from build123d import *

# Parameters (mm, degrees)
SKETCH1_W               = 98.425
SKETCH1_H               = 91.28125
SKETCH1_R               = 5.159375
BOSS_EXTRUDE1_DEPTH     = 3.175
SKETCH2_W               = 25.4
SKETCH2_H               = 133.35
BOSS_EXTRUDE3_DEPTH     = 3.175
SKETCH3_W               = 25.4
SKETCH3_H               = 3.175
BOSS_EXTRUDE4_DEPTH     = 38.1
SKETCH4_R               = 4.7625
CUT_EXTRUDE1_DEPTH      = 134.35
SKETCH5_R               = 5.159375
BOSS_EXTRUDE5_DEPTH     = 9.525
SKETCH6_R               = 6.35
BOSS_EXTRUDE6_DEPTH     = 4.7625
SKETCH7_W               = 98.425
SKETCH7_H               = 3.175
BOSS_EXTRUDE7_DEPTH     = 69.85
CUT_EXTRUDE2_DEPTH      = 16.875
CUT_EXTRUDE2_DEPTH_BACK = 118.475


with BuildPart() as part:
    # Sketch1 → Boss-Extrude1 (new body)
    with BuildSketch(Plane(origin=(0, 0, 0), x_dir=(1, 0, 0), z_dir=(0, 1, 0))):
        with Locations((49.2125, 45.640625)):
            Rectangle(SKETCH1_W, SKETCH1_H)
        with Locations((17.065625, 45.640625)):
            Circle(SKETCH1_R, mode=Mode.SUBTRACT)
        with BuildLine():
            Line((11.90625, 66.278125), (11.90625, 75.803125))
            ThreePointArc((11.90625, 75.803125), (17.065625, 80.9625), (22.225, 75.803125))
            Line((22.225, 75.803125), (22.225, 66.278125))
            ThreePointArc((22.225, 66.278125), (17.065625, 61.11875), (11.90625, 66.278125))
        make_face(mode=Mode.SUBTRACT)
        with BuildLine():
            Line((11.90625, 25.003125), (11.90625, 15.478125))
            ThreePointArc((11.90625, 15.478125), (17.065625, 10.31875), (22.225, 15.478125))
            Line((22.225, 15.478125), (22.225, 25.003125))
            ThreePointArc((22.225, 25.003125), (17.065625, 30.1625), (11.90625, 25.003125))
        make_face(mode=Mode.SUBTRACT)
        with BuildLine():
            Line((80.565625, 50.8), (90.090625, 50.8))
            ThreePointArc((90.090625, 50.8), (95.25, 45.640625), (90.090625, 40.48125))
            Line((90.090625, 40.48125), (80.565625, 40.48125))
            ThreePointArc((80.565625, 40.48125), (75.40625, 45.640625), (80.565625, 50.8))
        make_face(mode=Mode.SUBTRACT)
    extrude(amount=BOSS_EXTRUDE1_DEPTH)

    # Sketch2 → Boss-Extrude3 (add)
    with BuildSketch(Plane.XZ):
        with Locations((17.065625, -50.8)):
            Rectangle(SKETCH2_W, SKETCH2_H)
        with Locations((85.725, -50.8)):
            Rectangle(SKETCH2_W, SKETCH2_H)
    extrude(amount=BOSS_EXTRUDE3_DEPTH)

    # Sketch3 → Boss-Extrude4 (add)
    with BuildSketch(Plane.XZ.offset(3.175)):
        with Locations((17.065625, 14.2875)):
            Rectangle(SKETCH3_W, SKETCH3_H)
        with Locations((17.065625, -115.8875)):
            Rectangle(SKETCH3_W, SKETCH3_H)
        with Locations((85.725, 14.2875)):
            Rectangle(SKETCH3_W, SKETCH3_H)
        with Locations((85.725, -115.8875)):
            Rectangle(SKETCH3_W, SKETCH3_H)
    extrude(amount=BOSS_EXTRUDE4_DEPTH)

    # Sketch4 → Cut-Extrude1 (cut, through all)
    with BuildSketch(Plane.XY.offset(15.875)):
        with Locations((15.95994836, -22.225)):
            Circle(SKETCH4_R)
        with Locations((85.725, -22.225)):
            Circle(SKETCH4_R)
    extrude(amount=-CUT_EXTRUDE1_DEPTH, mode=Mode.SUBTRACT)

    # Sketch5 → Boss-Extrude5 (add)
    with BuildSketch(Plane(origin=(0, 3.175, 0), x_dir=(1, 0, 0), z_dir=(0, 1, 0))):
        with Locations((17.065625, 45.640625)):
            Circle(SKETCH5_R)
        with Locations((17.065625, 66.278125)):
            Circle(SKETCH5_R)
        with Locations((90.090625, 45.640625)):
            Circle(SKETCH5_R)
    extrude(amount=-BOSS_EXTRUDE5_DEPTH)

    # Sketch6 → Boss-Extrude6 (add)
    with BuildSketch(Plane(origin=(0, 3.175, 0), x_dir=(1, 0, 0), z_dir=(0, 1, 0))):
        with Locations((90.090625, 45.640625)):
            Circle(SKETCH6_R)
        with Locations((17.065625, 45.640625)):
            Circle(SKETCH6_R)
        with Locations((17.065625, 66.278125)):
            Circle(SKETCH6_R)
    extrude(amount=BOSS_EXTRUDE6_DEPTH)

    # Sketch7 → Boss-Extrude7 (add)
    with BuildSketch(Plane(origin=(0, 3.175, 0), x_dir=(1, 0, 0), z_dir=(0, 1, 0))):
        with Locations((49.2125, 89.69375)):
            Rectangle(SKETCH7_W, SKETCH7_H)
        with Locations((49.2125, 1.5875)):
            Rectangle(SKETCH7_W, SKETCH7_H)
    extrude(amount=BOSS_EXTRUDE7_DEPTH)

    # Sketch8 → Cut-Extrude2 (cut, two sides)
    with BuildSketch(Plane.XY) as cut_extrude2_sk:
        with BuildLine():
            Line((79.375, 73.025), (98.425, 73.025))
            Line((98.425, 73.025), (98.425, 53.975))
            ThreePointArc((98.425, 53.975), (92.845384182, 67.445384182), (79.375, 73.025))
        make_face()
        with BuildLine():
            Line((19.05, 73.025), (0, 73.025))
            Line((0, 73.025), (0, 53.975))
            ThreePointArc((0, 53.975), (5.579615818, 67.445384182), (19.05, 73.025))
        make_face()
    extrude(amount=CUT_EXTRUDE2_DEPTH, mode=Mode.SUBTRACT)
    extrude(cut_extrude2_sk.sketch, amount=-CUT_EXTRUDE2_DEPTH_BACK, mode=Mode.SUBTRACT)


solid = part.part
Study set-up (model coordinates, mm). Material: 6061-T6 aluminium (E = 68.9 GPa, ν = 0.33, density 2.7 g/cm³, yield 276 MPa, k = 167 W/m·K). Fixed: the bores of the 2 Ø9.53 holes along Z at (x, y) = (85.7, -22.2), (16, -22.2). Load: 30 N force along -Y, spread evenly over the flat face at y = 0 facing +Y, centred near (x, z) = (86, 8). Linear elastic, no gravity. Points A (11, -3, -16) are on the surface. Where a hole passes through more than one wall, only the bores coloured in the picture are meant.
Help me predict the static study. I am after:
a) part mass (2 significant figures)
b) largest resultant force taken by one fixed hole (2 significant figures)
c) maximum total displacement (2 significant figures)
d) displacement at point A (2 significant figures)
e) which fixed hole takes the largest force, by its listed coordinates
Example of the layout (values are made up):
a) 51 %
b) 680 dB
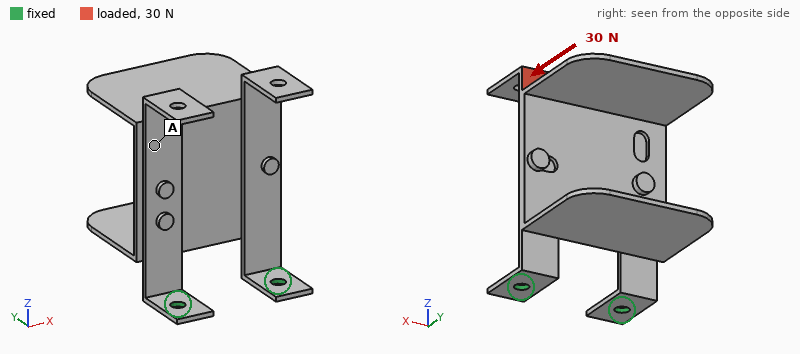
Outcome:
a) 280 g
b) 27 N
c) 2.1 mm
d) 1.3 mm
e) (85.7, -22.2)
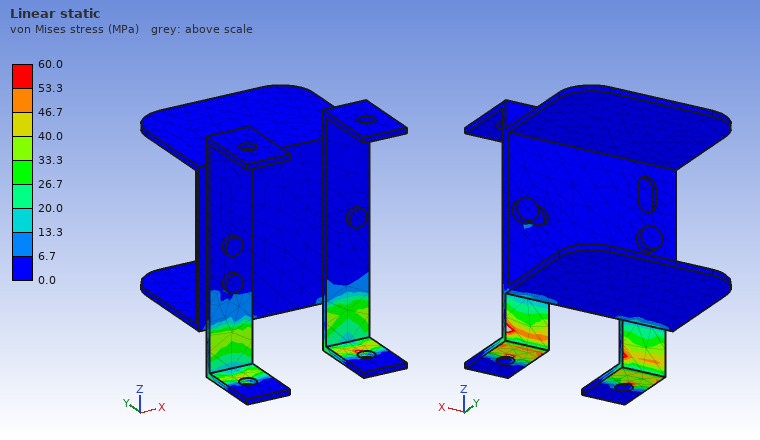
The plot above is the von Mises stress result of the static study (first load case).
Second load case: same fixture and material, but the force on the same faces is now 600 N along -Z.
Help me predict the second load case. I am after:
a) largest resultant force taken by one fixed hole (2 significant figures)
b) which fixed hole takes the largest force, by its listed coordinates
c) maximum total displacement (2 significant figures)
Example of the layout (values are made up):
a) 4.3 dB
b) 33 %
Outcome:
a) 570 N
b) (85.7, -22.2)
c) 2.0 mm
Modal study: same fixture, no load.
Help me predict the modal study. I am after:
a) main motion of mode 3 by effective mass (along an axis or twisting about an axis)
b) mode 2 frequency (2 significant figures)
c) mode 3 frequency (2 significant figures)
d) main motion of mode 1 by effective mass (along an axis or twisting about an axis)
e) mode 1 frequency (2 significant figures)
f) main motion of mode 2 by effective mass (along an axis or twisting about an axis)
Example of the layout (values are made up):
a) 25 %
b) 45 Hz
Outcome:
a) along X
b) 290 Hz
c) 380 Hz
d) along Y
e) 57 Hz
f) twisting about Z
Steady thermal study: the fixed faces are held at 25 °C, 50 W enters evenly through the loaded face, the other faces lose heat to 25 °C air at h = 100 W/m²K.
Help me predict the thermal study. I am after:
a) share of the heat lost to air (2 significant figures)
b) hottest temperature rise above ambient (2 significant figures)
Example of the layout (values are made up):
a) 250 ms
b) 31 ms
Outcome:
a) 96 %
b) 56 K
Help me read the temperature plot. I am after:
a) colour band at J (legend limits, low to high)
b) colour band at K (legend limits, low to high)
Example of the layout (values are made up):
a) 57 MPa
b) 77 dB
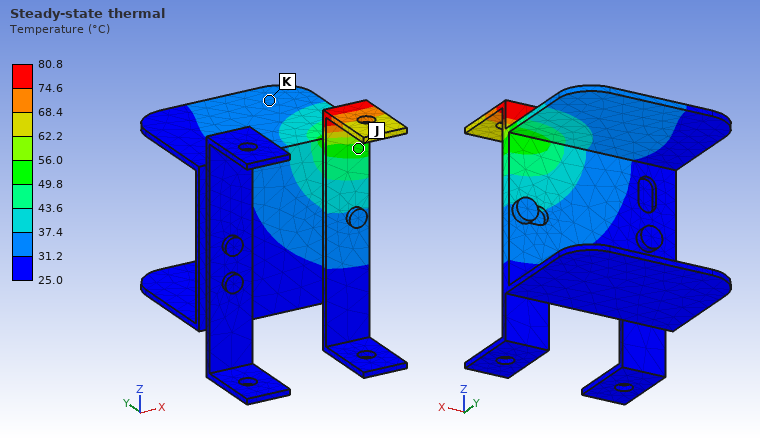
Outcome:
a) 49.8 to 56.0 °C
b) 31.2 to 37.4 °C
